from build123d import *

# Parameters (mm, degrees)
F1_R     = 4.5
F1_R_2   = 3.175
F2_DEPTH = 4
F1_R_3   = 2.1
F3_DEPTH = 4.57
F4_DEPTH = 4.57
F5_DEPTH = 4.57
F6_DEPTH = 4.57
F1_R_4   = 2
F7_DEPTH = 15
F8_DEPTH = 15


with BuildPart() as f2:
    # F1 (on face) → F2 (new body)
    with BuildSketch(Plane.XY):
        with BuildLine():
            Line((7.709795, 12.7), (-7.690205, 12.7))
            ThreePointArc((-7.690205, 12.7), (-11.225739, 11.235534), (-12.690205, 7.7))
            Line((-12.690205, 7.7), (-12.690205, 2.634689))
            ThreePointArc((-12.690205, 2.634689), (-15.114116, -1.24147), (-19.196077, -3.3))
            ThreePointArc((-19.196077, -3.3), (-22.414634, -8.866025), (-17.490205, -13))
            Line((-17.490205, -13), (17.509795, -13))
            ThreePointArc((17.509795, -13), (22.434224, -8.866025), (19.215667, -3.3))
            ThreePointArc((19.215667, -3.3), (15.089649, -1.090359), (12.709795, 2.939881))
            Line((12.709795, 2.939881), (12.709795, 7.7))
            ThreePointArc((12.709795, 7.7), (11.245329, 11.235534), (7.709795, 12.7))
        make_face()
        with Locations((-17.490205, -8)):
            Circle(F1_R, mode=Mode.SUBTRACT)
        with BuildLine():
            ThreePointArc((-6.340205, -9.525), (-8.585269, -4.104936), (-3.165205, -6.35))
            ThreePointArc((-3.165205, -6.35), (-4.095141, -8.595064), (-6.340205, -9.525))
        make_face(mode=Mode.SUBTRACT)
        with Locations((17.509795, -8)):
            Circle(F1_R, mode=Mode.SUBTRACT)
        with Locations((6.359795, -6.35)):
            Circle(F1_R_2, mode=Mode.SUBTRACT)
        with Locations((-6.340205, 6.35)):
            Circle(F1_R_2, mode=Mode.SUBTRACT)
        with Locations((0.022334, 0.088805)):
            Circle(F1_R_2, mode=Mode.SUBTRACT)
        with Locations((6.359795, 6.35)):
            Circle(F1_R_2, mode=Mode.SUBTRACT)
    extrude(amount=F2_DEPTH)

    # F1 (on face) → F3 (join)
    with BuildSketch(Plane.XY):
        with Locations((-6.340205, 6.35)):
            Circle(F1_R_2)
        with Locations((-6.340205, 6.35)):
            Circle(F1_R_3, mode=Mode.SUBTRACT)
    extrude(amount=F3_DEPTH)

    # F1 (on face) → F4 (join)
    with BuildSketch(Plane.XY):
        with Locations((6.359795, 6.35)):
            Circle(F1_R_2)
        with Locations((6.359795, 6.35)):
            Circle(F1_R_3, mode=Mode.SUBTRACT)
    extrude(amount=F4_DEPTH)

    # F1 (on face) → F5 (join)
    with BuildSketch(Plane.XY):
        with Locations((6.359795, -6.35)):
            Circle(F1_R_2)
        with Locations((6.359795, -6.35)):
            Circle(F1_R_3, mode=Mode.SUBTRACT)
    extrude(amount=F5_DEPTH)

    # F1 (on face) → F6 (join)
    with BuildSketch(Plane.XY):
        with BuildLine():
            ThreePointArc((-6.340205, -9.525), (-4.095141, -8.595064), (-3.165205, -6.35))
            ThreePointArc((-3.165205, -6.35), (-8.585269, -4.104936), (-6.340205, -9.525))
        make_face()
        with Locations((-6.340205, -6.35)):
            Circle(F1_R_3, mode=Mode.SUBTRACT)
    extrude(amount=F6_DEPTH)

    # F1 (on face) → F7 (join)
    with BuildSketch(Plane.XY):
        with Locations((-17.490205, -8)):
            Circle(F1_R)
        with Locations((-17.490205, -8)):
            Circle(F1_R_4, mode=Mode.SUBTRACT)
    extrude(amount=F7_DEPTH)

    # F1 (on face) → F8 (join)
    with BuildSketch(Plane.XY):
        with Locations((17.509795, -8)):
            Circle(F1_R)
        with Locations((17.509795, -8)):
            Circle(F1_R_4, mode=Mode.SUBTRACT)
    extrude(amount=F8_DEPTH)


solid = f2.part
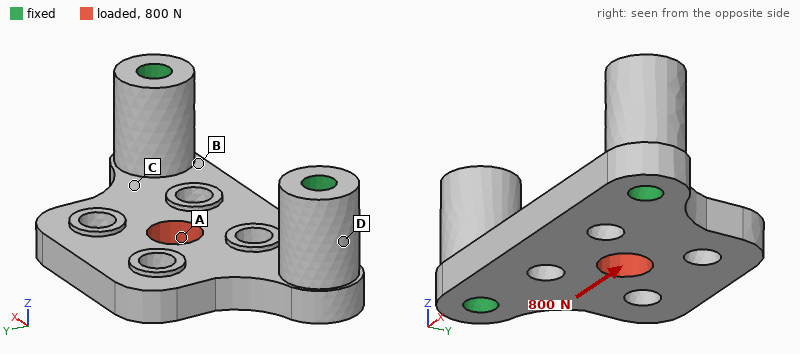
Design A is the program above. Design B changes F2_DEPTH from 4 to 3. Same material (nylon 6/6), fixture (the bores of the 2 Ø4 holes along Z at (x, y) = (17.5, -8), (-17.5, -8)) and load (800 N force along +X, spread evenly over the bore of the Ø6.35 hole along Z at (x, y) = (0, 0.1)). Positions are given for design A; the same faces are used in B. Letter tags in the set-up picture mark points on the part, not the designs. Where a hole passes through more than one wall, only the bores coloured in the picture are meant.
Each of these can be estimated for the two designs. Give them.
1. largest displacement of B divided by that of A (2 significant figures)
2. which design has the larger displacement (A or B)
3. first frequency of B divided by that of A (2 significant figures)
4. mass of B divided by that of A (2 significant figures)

1.3
B
0.79
0.86
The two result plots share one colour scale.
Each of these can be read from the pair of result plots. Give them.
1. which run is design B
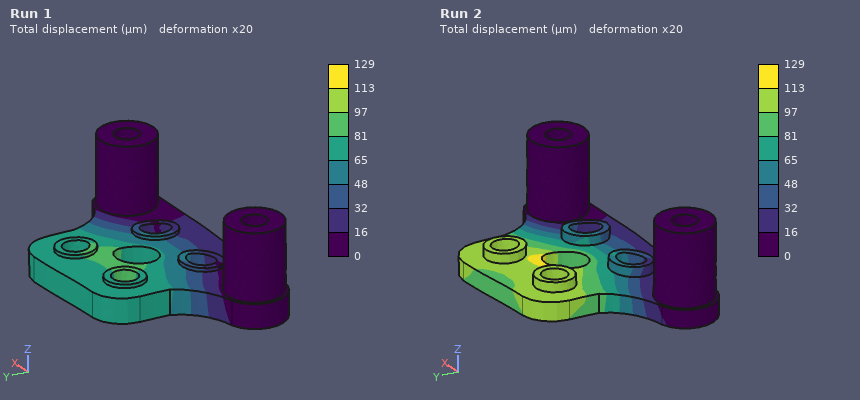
Run 2
